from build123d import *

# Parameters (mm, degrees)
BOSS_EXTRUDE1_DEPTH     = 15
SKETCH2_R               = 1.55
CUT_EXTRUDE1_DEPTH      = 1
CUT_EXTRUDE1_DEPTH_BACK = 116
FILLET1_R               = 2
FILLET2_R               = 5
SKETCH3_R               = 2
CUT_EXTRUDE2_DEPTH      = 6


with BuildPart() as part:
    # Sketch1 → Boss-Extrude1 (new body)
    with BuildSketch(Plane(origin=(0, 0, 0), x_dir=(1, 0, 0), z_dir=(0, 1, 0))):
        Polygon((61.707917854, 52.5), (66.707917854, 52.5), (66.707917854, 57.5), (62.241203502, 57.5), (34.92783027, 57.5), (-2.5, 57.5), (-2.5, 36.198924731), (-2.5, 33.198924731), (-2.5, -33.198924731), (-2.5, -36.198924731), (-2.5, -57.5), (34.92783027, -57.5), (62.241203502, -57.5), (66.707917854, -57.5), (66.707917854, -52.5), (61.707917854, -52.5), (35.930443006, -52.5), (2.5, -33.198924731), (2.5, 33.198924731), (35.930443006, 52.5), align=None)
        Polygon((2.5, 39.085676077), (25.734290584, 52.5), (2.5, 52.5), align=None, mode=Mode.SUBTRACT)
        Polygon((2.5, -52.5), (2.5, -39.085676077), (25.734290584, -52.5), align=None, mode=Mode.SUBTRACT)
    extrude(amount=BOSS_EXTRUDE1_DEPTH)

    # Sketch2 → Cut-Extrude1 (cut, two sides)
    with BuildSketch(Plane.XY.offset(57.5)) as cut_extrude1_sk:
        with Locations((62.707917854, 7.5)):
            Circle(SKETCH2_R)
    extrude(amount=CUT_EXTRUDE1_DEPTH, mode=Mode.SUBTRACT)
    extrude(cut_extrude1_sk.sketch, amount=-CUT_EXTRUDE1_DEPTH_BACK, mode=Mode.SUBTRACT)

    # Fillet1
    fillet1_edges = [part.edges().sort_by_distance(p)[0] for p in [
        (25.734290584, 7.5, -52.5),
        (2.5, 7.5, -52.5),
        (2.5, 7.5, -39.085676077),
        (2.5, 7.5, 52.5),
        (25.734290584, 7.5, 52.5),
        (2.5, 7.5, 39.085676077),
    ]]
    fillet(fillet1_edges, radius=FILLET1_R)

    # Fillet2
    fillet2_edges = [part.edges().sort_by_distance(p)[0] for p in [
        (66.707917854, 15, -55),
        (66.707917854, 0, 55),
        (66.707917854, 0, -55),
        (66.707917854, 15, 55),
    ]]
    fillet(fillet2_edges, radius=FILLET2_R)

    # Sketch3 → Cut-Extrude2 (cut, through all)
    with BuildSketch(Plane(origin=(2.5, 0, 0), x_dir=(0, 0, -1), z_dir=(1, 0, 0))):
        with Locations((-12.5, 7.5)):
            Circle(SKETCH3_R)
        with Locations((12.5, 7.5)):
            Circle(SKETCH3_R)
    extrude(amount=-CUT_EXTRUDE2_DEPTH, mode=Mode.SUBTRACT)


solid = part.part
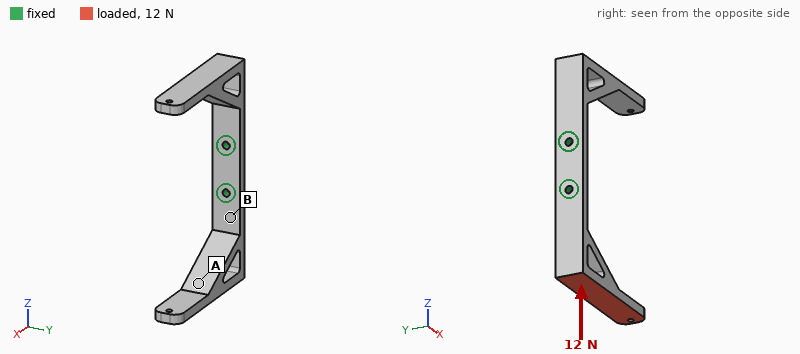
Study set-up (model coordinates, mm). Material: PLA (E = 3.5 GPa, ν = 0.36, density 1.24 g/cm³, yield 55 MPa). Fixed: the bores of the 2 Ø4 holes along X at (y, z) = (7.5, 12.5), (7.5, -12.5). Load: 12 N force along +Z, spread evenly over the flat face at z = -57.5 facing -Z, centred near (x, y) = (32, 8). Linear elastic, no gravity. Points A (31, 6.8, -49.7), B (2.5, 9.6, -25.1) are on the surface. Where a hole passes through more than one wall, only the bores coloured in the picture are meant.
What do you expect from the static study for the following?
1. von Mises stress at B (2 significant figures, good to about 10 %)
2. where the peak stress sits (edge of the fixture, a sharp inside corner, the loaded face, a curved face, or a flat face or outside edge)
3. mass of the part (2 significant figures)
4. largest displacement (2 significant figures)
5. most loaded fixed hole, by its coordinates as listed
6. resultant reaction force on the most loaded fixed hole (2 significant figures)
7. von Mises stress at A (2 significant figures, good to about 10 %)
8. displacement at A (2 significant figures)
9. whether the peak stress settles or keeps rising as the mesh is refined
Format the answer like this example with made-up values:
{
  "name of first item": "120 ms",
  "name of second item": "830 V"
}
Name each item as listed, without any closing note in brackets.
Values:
{
  "von Mises stress at B": "6.0 MPa",
  "where the peak stress sits": "edge of the fixture",
  "mass of the part": "29 g",
  "largest displacement": "1.3 mm",
  "most loaded fixed hole, by its coordinates as listed": "(7.5, -12.5)",
  "resultant reaction force on the most loaded fixed hole": "11 N",
  "von Mises stress at A": "0.71 MPa",
  "displacement at A": "0.66 mm",
  "whether the peak stress settles or keeps rising as the mesh is refined": "keeps rising"
}
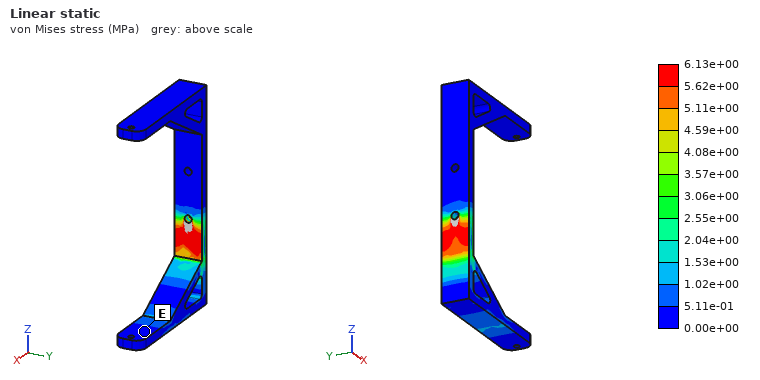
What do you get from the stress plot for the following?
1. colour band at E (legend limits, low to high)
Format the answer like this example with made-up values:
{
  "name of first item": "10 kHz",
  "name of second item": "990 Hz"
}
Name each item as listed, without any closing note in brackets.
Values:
{
  "colour band at E": "0.00e+00 to 5.11e-01 MPa"
}
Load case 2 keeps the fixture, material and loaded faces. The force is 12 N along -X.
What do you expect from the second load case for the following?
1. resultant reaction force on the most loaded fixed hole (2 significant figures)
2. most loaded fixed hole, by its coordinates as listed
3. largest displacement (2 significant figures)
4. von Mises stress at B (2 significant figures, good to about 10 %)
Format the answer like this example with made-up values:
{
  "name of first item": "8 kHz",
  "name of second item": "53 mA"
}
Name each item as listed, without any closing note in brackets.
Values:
{
  "resultant reaction force on the most loaded fixed hole": "15 N",
  "most loaded fixed hole, by its coordinates as listed": "(7.5, -12.5)",
  "largest displacement": "1.3 mm",
  "von Mises stress at B": "6.0 MPa"
}
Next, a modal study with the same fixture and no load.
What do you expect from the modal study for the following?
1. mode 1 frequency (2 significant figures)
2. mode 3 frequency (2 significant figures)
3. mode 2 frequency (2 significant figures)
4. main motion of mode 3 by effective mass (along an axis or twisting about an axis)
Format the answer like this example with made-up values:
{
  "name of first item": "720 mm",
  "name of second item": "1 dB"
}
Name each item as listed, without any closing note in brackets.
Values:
{
  "mode 1 frequency": "180 Hz",
  "mode 3 frequency": "260 Hz",
  "mode 2 frequency": "180 Hz",
  "main motion of mode 3 by effective mass": "along Y"
}
